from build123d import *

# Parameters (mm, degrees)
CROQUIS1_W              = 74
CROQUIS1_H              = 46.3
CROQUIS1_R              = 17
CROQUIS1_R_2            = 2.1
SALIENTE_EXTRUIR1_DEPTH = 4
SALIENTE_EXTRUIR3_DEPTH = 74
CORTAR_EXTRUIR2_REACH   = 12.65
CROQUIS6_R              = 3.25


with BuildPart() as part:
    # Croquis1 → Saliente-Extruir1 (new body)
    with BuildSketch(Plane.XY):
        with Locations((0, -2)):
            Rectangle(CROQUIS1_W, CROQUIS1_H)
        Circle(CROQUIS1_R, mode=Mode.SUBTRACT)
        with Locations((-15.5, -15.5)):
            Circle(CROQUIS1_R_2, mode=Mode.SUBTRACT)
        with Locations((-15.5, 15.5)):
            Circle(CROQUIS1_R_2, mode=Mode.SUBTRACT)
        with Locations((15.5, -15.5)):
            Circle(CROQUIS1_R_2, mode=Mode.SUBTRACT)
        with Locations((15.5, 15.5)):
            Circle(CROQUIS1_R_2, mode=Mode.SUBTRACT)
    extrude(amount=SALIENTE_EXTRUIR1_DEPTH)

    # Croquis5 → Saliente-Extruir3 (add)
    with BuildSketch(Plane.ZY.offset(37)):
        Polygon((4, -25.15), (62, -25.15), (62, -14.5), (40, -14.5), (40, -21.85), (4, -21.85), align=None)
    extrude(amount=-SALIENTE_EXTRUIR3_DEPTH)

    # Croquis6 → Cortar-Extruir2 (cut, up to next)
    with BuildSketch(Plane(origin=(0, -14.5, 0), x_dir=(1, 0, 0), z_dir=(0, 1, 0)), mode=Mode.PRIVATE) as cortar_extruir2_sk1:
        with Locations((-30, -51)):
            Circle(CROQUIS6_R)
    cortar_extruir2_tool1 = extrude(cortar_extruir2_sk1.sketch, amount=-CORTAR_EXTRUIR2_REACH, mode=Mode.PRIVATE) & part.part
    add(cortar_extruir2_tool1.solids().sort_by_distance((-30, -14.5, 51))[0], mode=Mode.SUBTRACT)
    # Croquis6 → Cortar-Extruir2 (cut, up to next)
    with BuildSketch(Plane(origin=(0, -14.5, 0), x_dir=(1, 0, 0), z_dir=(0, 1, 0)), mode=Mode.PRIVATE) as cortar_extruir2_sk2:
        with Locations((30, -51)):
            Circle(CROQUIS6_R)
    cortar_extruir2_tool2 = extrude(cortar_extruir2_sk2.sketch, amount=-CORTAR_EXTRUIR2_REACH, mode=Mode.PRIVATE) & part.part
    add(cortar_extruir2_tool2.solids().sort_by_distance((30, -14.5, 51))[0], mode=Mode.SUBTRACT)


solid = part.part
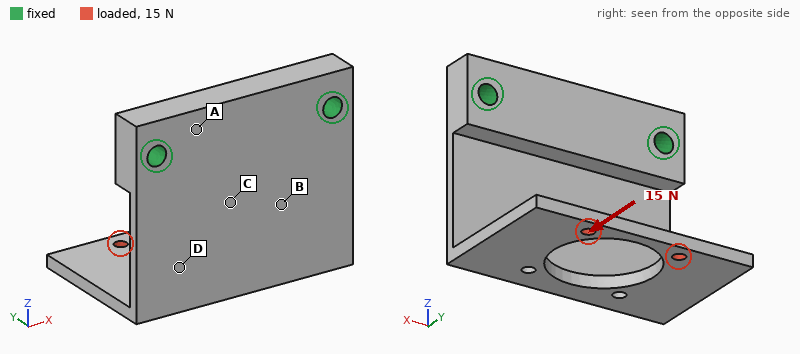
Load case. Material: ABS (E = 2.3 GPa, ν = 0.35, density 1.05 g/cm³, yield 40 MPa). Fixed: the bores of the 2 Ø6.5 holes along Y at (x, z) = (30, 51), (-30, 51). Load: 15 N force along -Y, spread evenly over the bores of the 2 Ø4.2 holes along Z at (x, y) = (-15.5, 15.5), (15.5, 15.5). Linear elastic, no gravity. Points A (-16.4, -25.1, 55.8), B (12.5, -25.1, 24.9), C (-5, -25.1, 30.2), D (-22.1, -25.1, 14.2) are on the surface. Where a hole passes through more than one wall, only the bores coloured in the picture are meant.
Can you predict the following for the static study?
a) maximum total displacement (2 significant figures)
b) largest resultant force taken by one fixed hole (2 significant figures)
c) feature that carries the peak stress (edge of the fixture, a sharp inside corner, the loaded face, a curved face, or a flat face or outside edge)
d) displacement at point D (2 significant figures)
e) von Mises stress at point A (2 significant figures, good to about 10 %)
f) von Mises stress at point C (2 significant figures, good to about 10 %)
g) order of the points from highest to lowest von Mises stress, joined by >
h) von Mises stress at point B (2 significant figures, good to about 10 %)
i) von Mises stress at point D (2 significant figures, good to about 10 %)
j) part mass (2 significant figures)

1.2 mm
7.5 N
a flat face or outside edge
0.33 mm
0.33 MPa
2.7 MPa
C > B > D > A
2.2 MPa
1.2 MPa
37 g
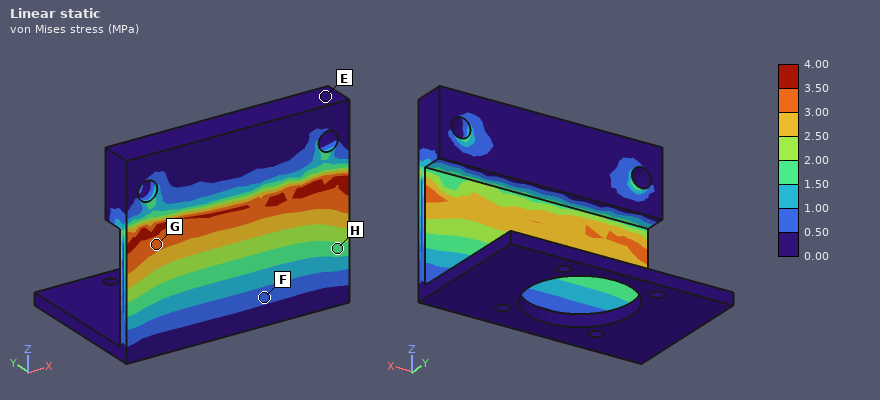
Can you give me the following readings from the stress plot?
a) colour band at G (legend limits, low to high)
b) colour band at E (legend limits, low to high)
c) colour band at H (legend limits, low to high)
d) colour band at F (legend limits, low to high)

3.00 to 3.50 MPa
0.00 to 0.50 MPa
1.50 to 2.00 MPa
0.50 to 1.00 MPa
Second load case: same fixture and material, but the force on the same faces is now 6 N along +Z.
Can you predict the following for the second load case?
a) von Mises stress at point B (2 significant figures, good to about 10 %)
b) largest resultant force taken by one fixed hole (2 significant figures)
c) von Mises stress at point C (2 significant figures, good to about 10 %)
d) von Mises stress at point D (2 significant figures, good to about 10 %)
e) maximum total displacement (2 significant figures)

1.5 MPa
3.2 N
1.5 MPa
1.5 MPa
1.1 mm
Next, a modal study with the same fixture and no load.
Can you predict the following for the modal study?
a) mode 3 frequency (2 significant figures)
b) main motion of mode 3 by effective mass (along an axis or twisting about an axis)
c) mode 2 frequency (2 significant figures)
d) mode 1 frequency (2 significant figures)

440 Hz
along Y
280 Hz
160 Hz
